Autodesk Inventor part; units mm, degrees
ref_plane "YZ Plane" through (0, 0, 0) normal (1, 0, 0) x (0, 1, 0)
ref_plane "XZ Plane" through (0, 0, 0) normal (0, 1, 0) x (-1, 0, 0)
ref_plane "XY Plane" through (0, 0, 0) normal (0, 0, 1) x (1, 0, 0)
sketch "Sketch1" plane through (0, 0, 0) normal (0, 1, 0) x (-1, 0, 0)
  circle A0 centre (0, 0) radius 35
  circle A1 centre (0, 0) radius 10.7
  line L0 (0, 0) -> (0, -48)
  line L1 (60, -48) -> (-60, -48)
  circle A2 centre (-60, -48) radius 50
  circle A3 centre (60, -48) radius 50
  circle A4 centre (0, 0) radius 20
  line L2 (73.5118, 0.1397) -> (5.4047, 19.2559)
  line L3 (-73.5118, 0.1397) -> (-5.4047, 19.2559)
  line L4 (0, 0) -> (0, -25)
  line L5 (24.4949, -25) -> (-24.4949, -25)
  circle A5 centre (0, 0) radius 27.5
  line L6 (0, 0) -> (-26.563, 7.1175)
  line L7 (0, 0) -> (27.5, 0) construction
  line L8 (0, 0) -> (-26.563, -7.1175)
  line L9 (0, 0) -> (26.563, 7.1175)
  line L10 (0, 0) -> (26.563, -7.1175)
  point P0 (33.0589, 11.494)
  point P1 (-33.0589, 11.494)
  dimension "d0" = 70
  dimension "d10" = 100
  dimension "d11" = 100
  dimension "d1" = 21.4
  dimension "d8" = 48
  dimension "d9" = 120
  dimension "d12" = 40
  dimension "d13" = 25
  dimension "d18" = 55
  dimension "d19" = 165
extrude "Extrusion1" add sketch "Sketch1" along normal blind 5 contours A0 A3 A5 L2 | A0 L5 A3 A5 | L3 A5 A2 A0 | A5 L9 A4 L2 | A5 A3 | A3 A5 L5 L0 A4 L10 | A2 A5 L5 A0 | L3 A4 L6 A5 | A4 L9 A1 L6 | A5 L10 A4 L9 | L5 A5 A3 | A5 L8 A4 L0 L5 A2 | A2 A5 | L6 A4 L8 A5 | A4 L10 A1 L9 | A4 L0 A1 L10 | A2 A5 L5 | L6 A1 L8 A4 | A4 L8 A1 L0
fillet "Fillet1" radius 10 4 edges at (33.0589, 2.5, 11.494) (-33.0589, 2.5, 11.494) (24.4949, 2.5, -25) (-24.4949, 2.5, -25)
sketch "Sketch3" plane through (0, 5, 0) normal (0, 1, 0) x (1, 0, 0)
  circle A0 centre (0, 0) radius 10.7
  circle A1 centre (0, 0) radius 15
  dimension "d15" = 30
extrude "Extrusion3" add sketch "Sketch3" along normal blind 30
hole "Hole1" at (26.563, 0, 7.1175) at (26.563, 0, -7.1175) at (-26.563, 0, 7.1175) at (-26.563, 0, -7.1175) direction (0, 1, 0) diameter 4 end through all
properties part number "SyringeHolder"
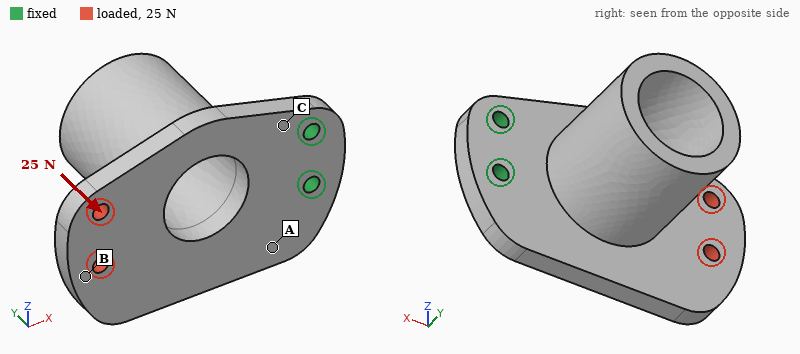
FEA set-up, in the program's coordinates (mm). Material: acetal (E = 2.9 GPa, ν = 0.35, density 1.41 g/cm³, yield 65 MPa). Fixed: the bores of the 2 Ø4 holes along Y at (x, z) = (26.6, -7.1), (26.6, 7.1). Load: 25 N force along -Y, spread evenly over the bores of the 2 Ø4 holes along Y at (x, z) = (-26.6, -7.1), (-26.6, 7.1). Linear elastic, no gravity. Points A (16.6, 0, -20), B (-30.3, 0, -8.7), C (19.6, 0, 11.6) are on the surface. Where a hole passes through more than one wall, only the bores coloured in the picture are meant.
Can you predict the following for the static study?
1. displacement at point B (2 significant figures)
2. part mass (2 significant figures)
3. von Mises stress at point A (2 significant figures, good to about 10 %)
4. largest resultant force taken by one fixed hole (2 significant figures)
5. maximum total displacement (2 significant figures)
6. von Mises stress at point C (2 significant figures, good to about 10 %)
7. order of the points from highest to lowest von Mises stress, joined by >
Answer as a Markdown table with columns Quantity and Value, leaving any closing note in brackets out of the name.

| Quantity | Value |
|---|---|
| displacement at point B | 0.91 mm |
| part mass | 31 g |
| von Mises stress at point A | 4.3 MPa |
| largest resultant force taken by one fixed hole | 16 N |
| maximum total displacement | 1.0 mm |
| von Mises stress at point C | 7.7 MPa |
| order of the points from highest to lowest von Mises stress, joined by > | C > A > B |
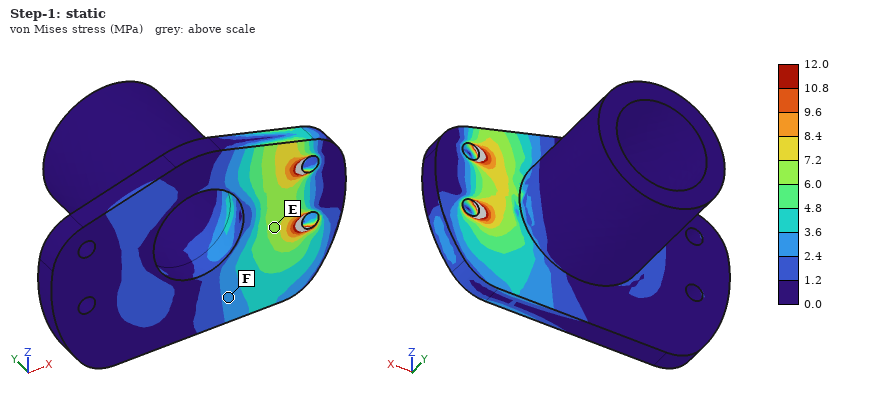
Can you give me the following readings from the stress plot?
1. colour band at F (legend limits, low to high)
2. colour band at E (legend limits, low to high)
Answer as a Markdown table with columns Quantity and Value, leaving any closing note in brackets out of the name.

| Quantity | Value |
|---|---|
| colour band at F | 2.4 to 3.6 MPa |
| colour band at E | 6.0 to 7.2 MPa |
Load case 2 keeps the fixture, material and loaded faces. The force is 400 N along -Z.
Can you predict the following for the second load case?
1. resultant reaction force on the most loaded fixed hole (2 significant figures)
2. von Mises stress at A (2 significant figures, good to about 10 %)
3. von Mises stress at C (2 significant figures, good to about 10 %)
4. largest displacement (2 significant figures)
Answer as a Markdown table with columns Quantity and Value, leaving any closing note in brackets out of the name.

| Quantity | Value |
|---|---|
| resultant reaction force on the most loaded fixed hole | 1.2 kN |
| von Mises stress at A | 7.1 MPa |
| von Mises stress at C | 13 MPa |
| largest displacement | 1.1 mm |
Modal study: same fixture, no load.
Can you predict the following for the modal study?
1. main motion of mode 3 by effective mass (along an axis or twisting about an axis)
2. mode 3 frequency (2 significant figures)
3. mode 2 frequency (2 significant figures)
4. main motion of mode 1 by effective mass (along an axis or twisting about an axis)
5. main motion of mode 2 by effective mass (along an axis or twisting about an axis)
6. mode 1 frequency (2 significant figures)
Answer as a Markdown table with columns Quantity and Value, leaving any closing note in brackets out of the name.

| Quantity | Value |
|---|---|
| main motion of mode 3 by effective mass | along Z |
| mode 3 frequency | 1100 Hz |
| mode 2 frequency | 690 Hz |
| main motion of mode 1 by effective mass | along Y |
| main motion of mode 2 by effective mass | along Z |
| mode 1 frequency | 270 Hz |
